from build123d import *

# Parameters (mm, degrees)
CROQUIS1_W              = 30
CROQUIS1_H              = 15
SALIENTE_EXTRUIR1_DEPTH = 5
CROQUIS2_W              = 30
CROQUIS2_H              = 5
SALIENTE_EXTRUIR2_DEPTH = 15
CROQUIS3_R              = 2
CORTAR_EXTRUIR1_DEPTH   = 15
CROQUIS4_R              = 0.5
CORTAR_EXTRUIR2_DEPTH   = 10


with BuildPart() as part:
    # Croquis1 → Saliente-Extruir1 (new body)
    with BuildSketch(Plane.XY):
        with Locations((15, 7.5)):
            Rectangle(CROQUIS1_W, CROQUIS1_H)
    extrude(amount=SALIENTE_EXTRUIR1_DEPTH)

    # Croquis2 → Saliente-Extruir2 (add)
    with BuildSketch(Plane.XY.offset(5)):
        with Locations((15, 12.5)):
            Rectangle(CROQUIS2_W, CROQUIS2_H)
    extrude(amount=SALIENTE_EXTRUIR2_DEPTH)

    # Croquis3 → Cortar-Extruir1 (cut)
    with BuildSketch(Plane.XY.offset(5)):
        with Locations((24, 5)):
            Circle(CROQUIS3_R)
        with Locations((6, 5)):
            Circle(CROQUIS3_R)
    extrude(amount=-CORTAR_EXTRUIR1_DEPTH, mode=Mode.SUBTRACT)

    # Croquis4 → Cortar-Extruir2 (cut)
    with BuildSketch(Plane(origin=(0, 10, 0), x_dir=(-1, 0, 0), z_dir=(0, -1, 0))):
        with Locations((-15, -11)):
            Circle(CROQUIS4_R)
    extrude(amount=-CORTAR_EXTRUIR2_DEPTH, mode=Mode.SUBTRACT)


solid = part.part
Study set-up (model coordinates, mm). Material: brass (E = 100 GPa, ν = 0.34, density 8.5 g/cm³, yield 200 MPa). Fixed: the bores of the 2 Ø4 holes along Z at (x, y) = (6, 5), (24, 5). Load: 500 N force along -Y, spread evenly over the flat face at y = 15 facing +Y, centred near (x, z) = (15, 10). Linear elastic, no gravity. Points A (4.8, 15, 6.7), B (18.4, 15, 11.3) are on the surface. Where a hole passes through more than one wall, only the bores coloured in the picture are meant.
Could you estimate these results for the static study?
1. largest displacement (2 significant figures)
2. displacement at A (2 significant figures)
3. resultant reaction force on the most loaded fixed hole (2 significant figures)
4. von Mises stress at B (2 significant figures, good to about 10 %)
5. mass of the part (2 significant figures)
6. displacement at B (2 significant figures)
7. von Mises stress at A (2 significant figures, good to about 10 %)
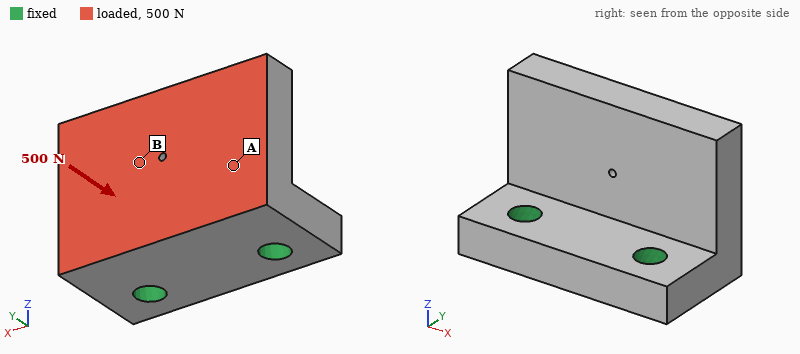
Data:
22 µm
7.0 µm
250 N
7.2 MPa
37 g
11 µm
17 MPa
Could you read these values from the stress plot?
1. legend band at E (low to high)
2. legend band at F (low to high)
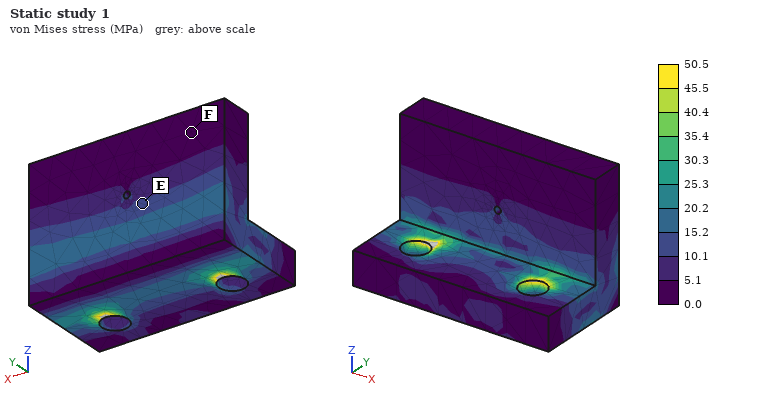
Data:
10.1 to 15.2 MPa
0.0 to 5.1 MPa
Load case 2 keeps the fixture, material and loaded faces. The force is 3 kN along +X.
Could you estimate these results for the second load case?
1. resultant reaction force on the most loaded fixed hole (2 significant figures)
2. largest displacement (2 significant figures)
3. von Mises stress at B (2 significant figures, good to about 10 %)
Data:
2.3 kN
24 µm
32 MPa
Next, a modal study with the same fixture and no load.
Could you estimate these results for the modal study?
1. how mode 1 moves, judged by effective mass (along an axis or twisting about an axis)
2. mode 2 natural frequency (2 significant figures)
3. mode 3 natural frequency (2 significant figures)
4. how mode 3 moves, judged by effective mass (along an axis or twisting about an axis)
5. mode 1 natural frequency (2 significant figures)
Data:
along Y
10 kHz
14 kHz
along X
5700 Hz
